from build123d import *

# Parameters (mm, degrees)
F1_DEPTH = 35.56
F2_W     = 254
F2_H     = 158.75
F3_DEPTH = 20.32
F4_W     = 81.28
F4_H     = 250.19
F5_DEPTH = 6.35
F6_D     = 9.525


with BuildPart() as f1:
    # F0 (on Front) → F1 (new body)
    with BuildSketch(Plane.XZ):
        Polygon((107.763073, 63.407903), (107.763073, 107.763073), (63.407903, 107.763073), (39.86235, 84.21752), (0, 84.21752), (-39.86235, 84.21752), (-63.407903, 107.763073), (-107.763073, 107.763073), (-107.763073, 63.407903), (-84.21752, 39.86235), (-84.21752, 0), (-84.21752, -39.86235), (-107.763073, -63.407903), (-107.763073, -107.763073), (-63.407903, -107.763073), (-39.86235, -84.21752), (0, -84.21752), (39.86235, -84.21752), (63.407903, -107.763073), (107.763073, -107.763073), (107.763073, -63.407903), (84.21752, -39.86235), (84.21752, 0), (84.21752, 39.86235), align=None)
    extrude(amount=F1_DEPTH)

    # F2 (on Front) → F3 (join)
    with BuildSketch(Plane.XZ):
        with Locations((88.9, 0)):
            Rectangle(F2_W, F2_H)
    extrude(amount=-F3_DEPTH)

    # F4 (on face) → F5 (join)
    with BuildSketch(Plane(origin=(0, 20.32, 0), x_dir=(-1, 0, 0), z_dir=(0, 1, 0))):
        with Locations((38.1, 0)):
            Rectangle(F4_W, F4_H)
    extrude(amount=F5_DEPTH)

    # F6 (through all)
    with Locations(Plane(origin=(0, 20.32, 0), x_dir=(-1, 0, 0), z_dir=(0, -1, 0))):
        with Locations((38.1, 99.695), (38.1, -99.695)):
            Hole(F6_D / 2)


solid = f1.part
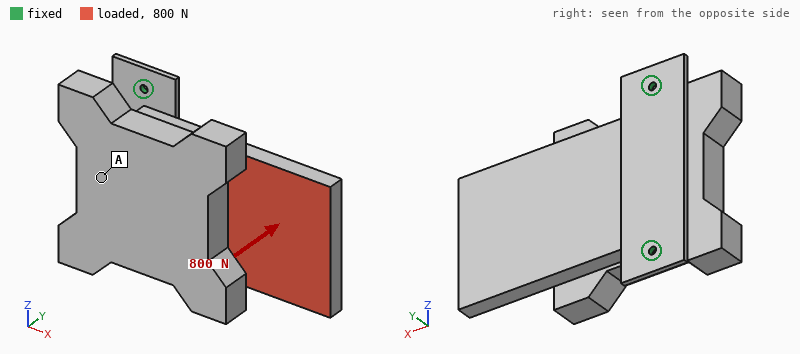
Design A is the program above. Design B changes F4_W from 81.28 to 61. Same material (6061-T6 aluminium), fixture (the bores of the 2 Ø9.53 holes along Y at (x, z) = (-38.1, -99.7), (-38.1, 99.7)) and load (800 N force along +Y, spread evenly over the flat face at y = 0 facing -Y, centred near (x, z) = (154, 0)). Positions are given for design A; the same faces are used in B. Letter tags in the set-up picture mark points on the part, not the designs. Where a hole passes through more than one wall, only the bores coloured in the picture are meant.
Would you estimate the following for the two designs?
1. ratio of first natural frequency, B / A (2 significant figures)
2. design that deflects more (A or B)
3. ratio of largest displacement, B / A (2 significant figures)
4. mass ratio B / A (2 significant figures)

0.94
B
1.1
0.99
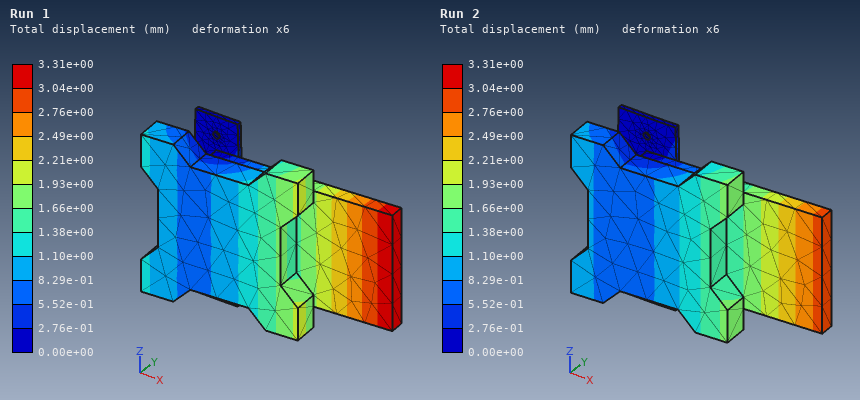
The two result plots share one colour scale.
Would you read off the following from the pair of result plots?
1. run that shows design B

Run 1
